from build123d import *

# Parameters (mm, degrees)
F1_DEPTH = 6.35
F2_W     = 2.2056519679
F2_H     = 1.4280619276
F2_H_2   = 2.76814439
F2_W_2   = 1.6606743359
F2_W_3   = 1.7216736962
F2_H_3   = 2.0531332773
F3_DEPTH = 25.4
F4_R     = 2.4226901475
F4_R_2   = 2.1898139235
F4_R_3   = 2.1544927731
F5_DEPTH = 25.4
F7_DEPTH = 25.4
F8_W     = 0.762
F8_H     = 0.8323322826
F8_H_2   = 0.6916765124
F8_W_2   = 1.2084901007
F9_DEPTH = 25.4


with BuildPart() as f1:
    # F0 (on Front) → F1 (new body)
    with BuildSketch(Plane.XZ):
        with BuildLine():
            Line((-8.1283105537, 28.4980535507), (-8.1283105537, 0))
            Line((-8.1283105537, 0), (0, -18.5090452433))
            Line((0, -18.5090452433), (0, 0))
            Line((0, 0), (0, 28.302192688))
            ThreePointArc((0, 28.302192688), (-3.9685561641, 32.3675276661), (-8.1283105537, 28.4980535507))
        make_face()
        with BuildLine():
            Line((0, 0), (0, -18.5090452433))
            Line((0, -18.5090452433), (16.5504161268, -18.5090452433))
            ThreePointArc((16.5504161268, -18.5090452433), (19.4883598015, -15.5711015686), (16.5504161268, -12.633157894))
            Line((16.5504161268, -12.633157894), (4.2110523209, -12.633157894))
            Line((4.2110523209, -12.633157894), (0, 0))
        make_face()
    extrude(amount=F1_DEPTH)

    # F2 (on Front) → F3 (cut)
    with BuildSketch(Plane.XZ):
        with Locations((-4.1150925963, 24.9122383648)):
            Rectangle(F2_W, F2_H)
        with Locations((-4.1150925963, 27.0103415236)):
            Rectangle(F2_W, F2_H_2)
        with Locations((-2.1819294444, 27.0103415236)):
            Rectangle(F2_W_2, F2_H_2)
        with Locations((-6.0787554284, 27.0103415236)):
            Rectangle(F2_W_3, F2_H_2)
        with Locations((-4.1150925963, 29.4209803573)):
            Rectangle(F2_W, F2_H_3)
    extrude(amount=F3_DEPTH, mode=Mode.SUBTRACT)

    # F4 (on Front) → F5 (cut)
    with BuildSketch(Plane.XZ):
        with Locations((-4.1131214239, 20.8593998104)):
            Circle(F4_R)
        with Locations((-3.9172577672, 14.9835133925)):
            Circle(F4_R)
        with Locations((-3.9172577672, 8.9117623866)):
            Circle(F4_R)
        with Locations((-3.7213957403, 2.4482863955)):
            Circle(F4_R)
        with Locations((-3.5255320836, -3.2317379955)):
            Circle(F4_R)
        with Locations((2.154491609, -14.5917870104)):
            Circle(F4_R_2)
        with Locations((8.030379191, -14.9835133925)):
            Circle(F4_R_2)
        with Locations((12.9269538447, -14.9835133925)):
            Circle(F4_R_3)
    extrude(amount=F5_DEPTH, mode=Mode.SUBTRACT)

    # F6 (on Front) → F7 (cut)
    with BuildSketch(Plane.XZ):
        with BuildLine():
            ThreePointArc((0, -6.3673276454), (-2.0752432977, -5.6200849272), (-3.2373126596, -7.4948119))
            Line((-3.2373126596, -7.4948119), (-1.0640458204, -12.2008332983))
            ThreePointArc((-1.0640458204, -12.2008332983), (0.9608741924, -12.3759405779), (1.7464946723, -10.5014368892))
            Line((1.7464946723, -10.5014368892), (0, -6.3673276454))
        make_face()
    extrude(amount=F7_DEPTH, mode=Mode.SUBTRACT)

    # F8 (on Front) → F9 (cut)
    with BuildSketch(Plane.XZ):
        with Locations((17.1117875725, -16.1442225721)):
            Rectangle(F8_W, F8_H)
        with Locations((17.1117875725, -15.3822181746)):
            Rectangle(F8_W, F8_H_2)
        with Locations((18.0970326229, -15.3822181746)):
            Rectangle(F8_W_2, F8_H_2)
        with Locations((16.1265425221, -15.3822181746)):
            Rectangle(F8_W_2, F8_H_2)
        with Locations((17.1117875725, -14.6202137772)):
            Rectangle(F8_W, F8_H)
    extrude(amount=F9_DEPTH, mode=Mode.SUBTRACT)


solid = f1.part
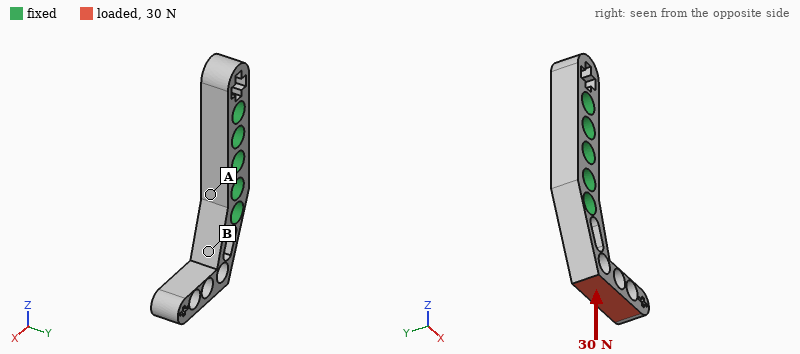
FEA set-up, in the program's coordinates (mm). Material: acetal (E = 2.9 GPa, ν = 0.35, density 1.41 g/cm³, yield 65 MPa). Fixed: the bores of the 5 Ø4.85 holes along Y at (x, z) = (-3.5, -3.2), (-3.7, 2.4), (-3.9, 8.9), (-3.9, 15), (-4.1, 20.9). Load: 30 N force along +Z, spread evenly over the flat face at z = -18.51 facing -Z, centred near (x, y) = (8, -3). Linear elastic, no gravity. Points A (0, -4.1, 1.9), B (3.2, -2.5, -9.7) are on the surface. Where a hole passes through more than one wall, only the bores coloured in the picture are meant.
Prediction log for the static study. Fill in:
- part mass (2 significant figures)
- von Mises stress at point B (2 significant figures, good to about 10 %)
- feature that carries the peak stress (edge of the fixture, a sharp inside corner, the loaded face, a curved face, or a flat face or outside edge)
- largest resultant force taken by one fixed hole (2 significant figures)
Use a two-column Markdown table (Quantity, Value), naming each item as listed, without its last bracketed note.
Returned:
| Quantity | Value |
|---|---|
| part mass | 2.5 g |
| von Mises stress at point B | 6.6 MPa |
| feature that carries the peak stress | a curved face |
| largest resultant force taken by one fixed hole | 19 N |
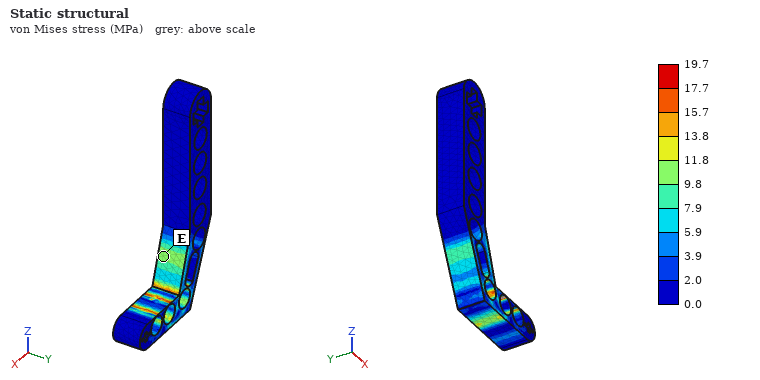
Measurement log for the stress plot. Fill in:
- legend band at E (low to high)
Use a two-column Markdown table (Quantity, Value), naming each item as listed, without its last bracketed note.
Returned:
| Quantity | Value |
|---|---|
| legend band at E | 9.8 to 11.8 MPa |
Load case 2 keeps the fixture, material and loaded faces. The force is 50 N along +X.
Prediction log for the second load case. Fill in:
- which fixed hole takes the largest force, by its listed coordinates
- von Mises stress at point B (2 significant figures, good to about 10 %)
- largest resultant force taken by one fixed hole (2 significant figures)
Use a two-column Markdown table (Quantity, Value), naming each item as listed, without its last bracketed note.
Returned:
| Quantity | Value |
|---|---|
| which fixed hole takes the largest force, by its listed coordinates | (-3.5, -3.2) |
| von Mises stress at point B | 6.3 MPa |
| largest resultant force taken by one fixed hole | 77 N |
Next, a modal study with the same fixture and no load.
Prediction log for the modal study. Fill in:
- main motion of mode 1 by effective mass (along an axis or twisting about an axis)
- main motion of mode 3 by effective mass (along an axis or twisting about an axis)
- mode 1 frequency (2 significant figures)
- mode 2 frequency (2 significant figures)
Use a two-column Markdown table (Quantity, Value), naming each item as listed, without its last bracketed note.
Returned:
| Quantity | Value |
|---|---|
| main motion of mode 1 by effective mass | along Y |
| main motion of mode 3 by effective mass | along X |
| mode 1 frequency | 1400 Hz |
| mode 2 frequency | 1700 Hz |
